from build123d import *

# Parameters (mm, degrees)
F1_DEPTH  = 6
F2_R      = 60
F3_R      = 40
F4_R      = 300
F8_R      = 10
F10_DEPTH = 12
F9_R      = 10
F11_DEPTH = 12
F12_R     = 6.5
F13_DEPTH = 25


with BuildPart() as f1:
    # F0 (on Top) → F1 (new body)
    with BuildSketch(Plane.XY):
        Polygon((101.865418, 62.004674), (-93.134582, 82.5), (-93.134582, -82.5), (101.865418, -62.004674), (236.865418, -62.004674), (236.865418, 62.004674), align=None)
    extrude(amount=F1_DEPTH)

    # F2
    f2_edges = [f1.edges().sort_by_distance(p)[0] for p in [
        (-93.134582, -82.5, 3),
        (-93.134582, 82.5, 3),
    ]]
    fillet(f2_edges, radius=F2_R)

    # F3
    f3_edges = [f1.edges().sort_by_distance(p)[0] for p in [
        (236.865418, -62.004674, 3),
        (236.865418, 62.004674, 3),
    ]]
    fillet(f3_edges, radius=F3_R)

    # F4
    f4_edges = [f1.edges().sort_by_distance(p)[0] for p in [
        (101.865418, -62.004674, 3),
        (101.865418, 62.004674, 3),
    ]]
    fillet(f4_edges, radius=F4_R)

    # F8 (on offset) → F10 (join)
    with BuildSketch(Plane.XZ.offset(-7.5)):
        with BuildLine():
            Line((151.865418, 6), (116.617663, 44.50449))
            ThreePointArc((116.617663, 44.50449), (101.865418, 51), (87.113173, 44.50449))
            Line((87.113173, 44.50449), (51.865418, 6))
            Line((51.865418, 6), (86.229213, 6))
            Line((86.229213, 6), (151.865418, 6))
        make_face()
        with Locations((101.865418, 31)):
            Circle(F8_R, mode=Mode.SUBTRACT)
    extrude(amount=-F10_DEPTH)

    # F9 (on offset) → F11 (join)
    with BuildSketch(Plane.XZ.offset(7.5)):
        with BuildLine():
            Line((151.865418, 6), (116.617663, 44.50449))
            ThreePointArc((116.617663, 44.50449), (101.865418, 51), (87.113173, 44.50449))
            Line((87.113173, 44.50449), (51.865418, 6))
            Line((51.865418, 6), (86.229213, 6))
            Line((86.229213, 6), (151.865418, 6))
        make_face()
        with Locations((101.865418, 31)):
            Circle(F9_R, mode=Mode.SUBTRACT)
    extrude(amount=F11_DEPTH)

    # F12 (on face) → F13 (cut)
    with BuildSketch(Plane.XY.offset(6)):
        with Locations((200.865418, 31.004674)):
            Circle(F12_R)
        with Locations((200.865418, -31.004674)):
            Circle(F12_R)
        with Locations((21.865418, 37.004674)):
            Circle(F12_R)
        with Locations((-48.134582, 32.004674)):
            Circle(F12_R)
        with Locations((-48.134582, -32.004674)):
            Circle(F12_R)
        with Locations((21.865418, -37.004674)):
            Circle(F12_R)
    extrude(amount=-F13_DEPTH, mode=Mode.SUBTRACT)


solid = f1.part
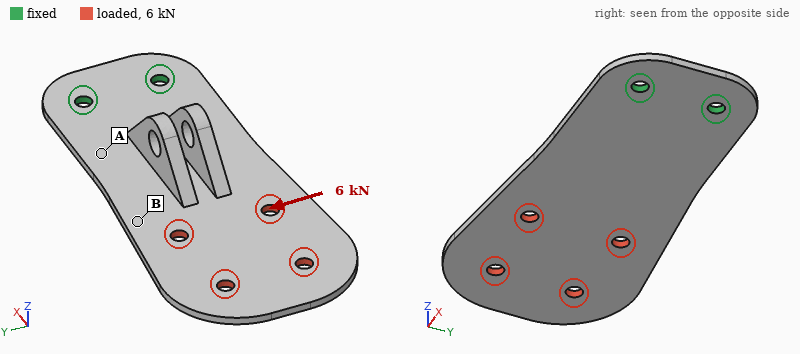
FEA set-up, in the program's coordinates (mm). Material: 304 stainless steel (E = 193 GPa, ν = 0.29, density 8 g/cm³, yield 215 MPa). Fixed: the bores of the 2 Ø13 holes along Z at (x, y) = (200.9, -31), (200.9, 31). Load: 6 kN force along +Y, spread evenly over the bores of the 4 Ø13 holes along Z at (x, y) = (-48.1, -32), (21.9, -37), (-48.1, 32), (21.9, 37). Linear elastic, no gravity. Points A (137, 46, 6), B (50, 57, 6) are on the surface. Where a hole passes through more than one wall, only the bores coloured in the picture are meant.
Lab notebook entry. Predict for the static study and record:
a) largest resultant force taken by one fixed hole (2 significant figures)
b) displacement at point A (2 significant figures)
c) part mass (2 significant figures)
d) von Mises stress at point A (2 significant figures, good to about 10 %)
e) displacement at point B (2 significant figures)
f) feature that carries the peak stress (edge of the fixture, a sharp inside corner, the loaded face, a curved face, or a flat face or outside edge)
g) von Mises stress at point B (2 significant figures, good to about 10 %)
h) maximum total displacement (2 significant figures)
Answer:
19 kN
0.041 mm
2.4 kg
43 MPa
0.11 mm
edge of the fixture
17 MPa
0.24 mm
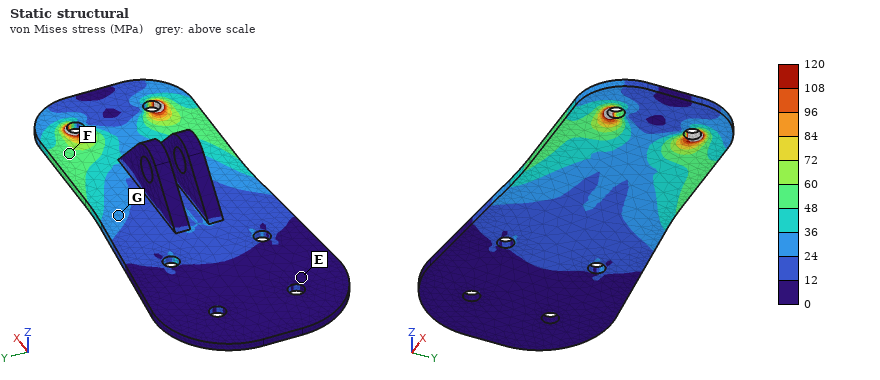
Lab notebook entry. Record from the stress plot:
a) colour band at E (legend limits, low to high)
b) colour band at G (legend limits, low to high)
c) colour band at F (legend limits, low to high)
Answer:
0 to 12 MPa
24 to 36 MPa
48 to 60 MPa
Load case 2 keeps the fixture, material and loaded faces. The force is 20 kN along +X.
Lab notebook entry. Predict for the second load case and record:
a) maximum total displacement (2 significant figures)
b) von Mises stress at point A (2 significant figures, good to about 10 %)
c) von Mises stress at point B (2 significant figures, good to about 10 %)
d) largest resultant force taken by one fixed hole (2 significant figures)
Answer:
0.14 mm
21 MPa
21 MPa
10 kN
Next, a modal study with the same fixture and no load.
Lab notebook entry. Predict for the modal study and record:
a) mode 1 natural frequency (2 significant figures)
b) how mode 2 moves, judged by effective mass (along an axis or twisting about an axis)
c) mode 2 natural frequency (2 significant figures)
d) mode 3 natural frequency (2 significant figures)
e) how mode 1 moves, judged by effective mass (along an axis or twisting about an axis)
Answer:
67 Hz
twisting about X
310 Hz
380 Hz
along Z
